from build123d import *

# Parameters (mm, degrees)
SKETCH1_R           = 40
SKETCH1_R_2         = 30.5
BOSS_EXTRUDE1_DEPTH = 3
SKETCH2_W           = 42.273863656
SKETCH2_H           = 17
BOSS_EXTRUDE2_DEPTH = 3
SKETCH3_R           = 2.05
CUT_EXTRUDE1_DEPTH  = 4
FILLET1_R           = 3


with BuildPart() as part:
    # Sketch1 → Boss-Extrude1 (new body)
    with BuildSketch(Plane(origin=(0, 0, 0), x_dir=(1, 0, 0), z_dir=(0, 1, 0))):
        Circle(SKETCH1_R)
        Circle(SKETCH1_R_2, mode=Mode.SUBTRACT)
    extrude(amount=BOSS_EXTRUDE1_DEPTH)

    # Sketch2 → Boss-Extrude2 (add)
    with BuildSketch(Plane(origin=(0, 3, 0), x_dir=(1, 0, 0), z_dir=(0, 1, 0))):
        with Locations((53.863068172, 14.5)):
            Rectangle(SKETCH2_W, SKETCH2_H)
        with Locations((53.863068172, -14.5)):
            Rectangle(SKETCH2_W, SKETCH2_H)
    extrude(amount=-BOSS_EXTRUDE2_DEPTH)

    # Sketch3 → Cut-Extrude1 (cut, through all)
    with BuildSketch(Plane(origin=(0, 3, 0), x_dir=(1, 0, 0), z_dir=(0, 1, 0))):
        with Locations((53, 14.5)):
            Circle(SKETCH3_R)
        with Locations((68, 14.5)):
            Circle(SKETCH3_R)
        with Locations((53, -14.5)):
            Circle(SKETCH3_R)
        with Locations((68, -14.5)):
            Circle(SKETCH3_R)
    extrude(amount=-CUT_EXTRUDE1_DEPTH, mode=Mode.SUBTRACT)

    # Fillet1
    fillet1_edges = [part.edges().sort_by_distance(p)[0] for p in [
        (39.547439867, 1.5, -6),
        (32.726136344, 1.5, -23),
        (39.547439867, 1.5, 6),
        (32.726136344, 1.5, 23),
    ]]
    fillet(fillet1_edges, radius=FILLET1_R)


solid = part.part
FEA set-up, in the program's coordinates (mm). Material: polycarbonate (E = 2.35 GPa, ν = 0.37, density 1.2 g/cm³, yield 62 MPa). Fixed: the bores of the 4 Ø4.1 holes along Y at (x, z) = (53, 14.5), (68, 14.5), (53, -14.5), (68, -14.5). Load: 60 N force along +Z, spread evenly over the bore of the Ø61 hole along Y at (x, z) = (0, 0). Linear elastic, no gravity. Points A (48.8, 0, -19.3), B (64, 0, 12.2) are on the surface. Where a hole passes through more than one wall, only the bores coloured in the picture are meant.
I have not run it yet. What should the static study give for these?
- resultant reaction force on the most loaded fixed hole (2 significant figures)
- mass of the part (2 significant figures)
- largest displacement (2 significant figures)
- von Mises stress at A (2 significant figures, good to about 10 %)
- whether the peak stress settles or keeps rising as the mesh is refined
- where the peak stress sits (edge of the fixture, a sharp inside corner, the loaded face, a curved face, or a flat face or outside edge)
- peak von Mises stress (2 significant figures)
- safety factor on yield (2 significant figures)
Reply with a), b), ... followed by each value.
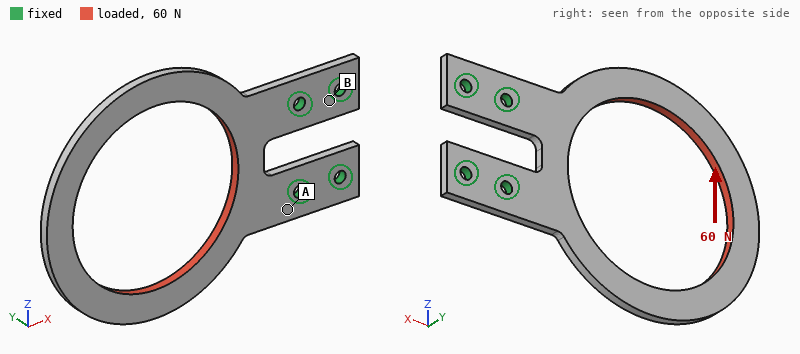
a) 80 N
b) 12 g
c) 1.4 mm
d) 2.8 MPa
e) settles
f) a curved face
g) 20 MPa
h) 3.1
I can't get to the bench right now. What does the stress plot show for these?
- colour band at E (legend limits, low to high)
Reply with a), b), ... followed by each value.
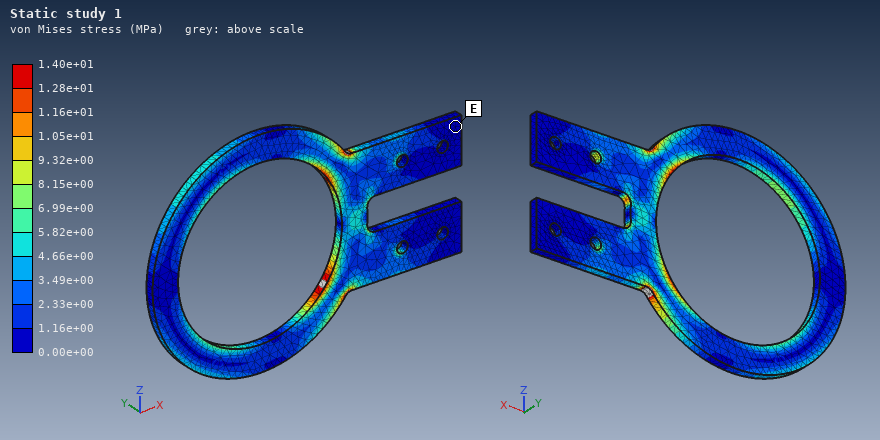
a) 0.00e+00 to 1.16e+00 MPa
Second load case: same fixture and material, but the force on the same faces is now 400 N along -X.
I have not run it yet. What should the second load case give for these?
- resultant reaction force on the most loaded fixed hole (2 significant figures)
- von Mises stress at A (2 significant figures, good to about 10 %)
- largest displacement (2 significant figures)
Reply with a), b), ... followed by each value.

a) 180 N
b) 6.8 MPa
c) 1.2 mm
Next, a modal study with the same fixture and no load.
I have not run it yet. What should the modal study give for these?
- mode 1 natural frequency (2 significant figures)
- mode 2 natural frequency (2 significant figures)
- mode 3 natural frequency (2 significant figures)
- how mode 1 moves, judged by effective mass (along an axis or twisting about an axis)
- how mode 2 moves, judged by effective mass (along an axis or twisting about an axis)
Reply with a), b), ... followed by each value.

a) 73 Hz
b) 180 Hz
c) 390 Hz
d) along Y
e) twisting about X
